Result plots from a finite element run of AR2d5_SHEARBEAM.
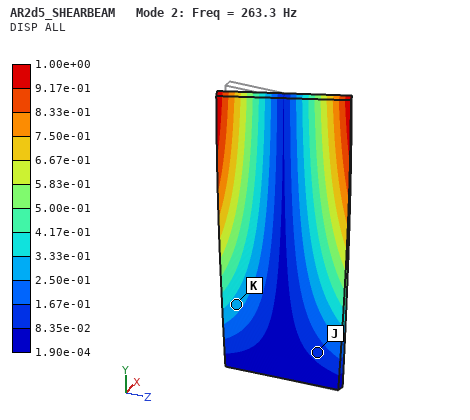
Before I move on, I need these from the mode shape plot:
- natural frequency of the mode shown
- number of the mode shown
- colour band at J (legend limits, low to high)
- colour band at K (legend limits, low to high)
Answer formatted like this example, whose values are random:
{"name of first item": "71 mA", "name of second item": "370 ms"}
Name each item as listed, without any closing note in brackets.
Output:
{"natural frequency of the mode shown": "263.3 Hz", "number of the mode shown": "2", "colour band at J": "8.35e-02 to 1.67e-01", "colour band at K": "2.50e-01 to 3.33e-01"}
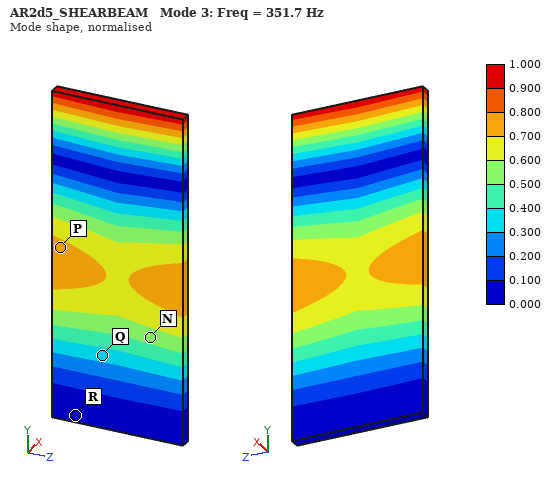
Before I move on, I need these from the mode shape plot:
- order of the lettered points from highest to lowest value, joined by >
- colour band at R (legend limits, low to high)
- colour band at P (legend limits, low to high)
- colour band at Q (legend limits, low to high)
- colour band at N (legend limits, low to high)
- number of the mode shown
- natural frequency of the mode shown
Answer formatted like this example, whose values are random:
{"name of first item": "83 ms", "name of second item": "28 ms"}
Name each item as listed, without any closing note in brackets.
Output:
{"order of the lettered points from highest to lowest value, joined by >": "P > N > Q > R", "colour band at R": "0.000 to 0.100", "colour band at P": "0.700 to 0.800", "colour band at Q": "0.300 to 0.400", "colour band at N": "0.500 to 0.600", "number of the mode shown": "3", "natural frequency of the mode shown": "351.7 Hz"}
